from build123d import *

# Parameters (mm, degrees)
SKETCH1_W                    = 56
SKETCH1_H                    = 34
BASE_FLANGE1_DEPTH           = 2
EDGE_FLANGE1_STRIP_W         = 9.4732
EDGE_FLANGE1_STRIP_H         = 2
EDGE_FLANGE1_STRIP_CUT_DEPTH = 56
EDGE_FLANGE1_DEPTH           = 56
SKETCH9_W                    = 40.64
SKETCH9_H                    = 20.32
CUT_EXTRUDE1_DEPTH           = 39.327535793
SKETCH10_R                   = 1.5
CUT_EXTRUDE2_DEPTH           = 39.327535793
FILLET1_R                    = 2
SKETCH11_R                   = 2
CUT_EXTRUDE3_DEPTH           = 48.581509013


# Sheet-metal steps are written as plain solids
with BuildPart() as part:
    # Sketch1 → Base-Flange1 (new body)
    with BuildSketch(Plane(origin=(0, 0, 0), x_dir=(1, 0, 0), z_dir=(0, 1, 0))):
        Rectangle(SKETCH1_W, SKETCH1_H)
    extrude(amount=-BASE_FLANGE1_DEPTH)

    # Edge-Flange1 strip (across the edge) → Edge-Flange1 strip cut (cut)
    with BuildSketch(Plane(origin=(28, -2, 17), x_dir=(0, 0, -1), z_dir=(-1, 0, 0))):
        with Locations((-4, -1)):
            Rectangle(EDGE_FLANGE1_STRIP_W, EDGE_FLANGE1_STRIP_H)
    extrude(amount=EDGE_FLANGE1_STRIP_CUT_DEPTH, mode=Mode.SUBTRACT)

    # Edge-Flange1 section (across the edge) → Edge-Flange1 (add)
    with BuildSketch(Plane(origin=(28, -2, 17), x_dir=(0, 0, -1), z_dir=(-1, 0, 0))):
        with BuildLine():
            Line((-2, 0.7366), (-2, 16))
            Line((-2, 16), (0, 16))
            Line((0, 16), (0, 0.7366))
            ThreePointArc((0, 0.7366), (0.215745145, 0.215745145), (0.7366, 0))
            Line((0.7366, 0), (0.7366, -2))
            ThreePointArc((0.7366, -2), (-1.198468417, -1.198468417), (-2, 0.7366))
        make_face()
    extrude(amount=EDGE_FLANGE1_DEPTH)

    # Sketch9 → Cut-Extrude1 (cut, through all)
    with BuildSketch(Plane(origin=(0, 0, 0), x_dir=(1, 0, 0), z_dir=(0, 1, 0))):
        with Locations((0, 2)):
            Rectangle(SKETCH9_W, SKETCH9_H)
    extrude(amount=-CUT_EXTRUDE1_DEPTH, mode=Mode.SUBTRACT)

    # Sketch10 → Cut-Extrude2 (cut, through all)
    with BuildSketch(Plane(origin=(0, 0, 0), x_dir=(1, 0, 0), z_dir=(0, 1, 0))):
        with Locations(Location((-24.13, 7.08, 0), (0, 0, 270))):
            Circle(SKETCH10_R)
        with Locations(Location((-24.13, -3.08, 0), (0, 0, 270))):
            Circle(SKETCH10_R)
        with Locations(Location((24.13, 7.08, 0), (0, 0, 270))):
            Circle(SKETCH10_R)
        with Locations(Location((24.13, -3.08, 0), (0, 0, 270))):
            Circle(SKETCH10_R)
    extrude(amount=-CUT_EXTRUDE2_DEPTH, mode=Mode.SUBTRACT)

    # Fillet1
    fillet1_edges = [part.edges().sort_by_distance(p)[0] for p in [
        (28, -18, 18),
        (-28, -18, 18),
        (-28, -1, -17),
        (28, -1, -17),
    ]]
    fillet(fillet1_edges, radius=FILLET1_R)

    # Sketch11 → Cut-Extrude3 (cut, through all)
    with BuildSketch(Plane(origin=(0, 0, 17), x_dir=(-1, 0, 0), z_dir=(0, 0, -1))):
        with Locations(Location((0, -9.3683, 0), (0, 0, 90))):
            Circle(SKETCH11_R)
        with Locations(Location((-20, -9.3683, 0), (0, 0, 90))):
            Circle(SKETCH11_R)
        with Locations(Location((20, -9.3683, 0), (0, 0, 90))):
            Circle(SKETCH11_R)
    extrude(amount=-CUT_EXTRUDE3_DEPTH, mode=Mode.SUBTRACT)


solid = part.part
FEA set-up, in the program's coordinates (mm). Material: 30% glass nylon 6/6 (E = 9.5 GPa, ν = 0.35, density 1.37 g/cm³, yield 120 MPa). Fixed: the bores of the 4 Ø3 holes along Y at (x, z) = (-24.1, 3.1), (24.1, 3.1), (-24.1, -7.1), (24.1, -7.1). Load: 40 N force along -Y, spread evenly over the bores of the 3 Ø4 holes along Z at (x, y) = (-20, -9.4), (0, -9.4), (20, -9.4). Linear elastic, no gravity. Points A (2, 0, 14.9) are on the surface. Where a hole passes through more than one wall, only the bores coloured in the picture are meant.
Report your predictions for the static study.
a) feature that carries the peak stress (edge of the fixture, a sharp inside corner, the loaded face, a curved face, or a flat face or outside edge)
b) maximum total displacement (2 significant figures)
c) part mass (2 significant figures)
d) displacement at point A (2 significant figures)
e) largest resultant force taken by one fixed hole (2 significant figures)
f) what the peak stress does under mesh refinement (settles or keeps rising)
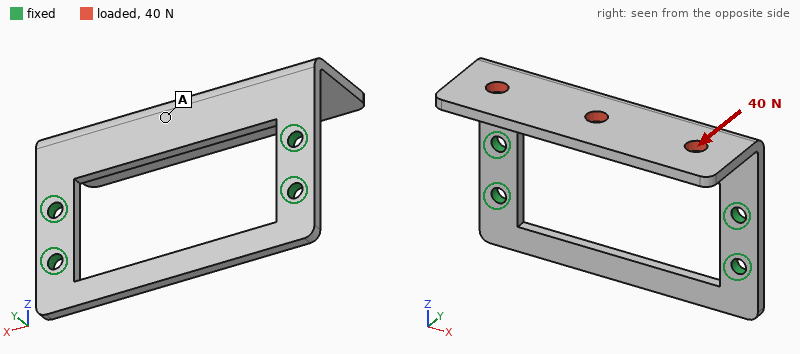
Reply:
edge of the fixture
0.69 mm
5.4 g
0.25 mm
21 N
keeps rising
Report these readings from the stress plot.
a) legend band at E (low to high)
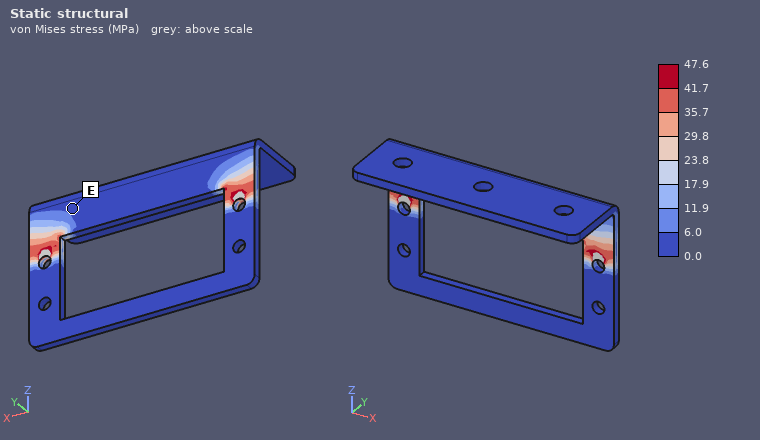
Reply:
0.0 to 6.0 MPa
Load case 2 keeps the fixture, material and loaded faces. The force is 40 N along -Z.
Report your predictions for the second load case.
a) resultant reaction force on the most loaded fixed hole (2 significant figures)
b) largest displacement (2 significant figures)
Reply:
22 N
0.73 mm
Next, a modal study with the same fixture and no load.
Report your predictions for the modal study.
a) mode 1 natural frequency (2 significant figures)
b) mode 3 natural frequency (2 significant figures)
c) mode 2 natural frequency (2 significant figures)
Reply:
720 Hz
2100 Hz
1600 Hz
